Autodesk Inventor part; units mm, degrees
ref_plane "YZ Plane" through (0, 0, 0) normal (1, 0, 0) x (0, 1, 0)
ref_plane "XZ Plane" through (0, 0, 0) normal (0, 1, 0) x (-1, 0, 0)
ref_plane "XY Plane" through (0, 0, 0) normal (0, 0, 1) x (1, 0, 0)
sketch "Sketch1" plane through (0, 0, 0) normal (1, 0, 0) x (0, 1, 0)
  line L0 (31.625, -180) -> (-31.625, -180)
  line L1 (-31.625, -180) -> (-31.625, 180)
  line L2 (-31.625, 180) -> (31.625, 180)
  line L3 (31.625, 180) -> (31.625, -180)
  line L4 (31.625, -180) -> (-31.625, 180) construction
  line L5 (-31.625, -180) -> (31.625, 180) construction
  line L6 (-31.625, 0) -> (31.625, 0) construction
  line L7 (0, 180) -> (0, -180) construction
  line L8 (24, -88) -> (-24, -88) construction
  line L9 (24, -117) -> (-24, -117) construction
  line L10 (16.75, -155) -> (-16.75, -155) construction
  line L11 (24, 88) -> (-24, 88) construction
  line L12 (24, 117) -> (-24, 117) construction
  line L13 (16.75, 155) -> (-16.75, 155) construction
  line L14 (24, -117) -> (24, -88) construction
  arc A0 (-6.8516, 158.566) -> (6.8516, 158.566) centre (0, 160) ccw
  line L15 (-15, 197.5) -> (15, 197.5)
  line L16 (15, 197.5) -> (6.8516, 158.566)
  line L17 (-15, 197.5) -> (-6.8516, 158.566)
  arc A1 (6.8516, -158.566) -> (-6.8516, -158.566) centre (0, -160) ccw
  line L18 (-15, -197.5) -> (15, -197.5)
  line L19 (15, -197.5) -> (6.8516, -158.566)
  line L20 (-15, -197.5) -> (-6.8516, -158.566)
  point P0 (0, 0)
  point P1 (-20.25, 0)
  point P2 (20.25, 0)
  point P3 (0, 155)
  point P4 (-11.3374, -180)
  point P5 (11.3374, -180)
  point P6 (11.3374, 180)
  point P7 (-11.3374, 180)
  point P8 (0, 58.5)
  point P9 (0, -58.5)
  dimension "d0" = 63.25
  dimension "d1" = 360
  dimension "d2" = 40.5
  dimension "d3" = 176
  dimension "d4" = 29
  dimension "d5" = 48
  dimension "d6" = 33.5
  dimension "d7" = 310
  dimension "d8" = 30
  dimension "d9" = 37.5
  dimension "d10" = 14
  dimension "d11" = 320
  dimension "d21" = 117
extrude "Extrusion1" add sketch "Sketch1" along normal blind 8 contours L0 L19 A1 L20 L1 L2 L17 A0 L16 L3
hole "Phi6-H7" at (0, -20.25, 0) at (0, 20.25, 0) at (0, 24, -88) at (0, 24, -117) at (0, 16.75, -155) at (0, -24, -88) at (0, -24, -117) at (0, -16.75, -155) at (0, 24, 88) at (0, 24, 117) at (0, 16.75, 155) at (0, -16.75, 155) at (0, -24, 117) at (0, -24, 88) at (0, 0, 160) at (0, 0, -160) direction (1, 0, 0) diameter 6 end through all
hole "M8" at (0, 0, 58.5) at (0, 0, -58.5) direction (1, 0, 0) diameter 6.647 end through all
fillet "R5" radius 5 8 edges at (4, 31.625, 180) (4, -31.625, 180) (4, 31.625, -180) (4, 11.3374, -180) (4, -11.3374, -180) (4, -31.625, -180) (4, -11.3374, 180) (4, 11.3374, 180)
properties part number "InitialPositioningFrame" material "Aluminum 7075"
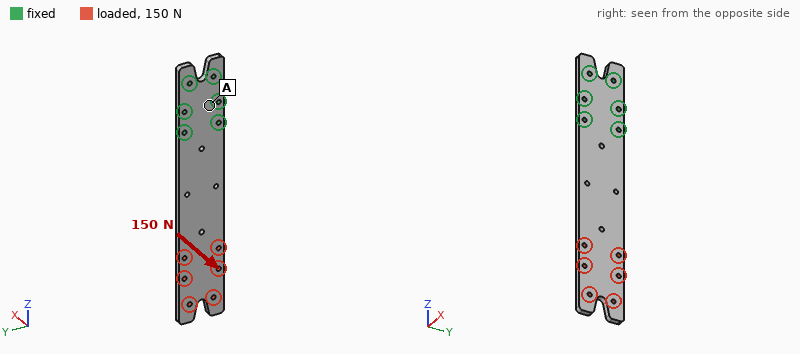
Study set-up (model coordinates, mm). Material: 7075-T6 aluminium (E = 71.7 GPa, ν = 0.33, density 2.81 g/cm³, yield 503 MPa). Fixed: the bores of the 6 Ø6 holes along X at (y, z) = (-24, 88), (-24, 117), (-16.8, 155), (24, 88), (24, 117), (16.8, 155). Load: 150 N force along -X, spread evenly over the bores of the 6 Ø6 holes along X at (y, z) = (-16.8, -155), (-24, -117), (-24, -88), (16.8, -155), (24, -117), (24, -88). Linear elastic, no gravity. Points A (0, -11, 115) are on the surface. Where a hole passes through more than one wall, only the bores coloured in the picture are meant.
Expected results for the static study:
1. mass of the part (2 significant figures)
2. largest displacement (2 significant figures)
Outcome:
480 g
3.5 mm
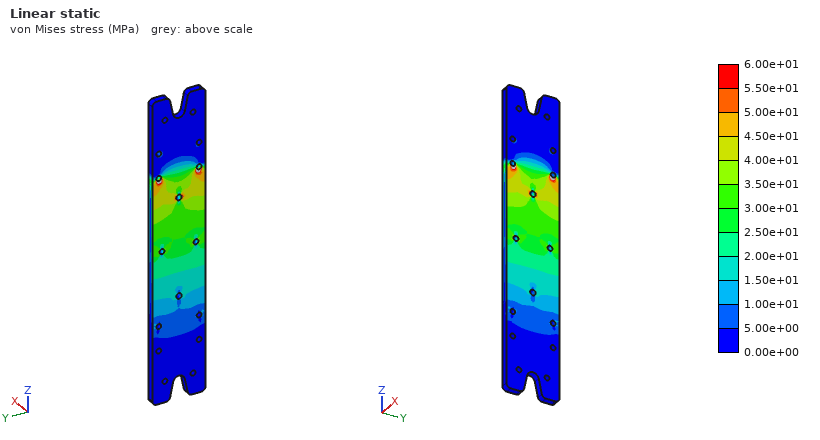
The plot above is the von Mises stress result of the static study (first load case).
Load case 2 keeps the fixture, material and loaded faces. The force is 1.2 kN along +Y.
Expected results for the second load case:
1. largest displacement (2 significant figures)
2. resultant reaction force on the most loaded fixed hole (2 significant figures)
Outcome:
0.47 mm
4.7 kN
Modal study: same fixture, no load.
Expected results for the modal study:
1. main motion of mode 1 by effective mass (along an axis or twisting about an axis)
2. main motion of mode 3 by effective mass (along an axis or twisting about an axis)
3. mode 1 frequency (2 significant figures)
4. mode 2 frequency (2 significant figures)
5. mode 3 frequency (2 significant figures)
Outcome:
along X
along Y
95 Hz
580 Hz
720 Hz
